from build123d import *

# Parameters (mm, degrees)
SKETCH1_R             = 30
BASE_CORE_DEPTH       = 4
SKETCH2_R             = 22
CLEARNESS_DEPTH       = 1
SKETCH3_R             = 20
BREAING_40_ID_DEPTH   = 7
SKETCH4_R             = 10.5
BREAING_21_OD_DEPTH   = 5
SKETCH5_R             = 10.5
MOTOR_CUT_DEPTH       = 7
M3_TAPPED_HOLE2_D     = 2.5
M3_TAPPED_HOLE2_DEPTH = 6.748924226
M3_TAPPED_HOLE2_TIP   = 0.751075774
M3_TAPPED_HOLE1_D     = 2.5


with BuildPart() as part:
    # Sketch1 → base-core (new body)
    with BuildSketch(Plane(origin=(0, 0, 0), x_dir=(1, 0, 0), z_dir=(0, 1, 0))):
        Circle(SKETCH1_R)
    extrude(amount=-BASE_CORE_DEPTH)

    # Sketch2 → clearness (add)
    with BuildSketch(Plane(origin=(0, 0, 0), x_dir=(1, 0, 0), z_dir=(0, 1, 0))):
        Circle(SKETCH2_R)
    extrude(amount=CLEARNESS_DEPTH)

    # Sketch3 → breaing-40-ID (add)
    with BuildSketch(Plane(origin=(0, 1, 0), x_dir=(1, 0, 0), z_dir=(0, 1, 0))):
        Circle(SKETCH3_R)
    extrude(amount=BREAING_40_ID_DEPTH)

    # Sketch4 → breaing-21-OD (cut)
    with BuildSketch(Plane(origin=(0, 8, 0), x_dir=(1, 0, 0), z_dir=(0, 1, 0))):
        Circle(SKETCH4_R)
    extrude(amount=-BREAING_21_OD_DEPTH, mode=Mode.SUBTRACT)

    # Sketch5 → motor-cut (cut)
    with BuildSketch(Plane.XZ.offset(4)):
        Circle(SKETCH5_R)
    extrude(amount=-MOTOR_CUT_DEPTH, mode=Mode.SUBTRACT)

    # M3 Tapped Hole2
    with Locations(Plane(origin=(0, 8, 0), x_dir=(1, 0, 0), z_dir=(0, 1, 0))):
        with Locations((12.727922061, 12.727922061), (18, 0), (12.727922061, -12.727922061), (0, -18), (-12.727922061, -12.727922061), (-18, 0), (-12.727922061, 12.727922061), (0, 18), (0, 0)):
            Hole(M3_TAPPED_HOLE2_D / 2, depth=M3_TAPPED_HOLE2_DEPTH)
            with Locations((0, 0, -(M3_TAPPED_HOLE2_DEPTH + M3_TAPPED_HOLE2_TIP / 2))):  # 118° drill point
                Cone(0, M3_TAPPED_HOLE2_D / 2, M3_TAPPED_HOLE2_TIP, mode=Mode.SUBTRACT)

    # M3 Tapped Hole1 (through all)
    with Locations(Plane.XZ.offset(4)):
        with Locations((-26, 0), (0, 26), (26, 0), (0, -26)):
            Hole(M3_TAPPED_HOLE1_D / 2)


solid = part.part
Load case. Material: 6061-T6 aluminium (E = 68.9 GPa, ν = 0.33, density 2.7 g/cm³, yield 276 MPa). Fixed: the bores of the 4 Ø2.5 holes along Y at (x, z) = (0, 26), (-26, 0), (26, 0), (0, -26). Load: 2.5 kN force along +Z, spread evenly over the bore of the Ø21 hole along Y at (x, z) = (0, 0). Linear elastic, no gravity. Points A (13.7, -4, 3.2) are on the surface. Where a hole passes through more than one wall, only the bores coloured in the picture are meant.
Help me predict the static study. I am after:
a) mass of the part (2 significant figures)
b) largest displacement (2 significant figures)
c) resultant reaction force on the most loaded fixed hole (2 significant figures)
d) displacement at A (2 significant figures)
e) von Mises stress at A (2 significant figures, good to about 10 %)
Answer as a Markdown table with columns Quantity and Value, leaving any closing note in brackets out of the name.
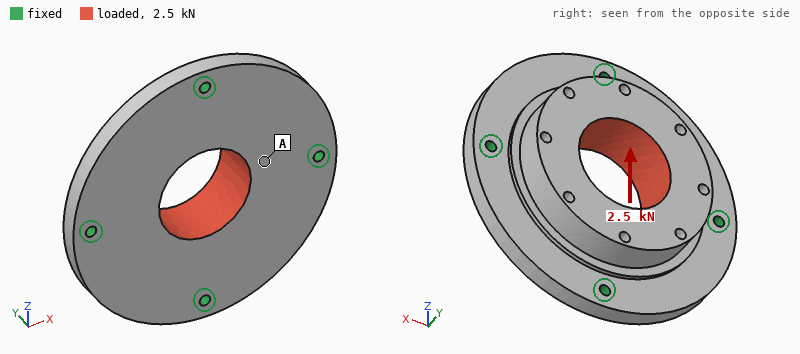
| Quantity | Value |
|---|---|
| mass of the part | 46 g |
| largest displacement | 4.3 µm |
| resultant reaction force on the most loaded fixed hole | 770 N |
| displacement at A | 2.6 µm |
| von Mises stress at A | 3.8 MPa |
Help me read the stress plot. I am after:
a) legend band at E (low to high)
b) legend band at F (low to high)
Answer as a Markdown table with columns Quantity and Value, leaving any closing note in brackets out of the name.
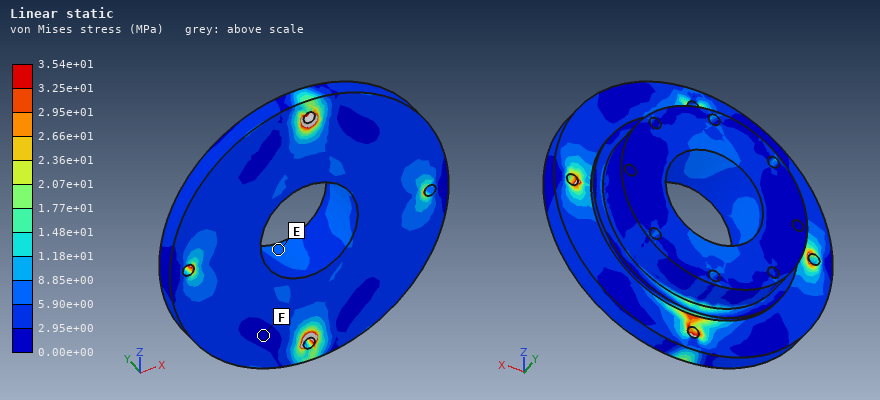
| Quantity | Value |
|---|---|
| legend band at E | 5.90e+00 to 8.85e+00 MPa |
| legend band at F | 0.00e+00 to 2.95e+00 MPa |
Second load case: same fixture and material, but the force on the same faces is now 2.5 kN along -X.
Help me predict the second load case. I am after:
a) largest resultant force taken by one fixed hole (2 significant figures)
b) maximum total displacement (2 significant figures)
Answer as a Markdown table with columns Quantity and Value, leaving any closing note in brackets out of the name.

| Quantity | Value |
|---|---|
| largest resultant force taken by one fixed hole | 770 N |
| maximum total displacement | 4.3 µm |
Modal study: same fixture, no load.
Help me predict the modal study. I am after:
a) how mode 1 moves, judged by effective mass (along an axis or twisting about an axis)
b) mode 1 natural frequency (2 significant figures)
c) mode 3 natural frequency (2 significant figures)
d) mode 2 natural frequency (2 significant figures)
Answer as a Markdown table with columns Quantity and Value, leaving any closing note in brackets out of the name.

| Quantity | Value |
|---|---|
| how mode 1 moves, judged by effective mass | along Y |
| mode 1 natural frequency | 13 kHz |
| mode 3 natural frequency | 14 kHz |
| mode 2 natural frequency | 14 kHz |
